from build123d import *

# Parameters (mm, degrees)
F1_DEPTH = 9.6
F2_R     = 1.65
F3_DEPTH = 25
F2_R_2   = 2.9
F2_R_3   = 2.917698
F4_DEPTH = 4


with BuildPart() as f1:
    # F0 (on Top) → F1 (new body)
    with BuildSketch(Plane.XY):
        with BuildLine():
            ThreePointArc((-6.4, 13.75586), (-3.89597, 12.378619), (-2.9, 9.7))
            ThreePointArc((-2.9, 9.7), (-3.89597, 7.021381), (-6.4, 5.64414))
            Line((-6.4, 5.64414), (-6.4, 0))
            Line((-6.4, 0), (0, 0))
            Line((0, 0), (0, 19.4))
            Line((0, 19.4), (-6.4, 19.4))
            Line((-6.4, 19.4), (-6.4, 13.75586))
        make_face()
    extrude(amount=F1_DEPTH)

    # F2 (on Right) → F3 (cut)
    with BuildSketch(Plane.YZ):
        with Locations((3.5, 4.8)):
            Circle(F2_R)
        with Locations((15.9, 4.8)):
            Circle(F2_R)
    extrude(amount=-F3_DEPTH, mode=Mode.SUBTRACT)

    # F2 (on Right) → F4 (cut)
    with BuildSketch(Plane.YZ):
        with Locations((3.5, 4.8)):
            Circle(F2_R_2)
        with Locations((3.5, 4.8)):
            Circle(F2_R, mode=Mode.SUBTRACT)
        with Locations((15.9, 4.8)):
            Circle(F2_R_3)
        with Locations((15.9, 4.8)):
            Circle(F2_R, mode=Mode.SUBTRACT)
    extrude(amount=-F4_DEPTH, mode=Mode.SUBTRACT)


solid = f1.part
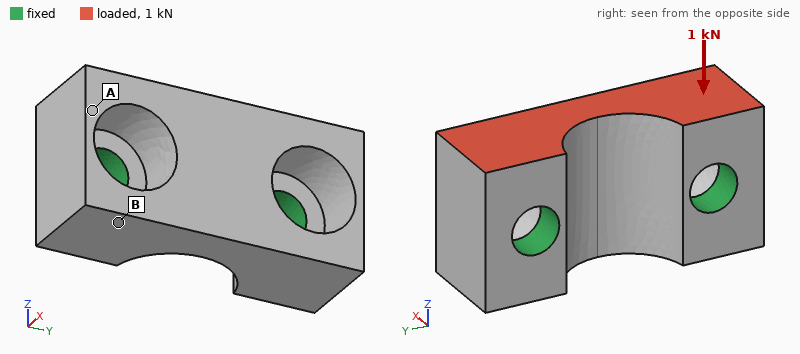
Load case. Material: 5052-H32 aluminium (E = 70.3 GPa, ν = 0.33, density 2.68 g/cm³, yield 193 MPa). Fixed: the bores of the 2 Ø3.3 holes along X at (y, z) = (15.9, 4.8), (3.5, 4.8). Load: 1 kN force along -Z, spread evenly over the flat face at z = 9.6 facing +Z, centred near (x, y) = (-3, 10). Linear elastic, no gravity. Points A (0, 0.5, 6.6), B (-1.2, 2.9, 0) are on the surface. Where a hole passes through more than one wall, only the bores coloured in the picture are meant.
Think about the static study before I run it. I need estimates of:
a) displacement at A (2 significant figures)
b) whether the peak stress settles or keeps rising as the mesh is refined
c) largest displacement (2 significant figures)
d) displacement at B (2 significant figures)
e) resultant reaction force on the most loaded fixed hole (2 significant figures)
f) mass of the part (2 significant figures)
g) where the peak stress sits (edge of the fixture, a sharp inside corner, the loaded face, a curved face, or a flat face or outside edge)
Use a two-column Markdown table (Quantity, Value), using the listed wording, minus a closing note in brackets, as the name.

| Quantity | Value |
|---|---|
| displacement at A | 7.3 µm |
| whether the peak stress settles or keeps rising as the mesh is refined | keeps rising |
| largest displacement | 11 µm |
| displacement at B | 6.2 µm |
| resultant reaction force on the most loaded fixed hole | 500 N |
| mass of the part | 2.0 g |
| where the peak stress sits | edge of the fixture |
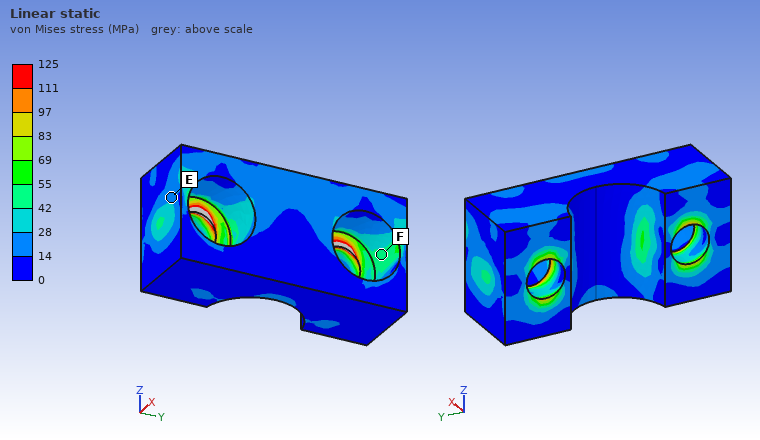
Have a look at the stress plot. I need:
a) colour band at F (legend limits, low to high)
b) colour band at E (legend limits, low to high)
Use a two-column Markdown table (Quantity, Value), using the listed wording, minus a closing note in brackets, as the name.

| Quantity | Value |
|---|---|
| colour band at F | 42 to 55 MPa |
| colour band at E | 14 to 28 MPa |
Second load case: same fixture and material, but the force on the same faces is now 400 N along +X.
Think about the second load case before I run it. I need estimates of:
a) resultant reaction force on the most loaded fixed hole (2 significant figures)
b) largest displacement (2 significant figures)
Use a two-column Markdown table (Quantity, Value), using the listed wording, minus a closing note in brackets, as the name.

| Quantity | Value |
|---|---|
| resultant reaction force on the most loaded fixed hole | 200 N |
| largest displacement | 7.2 µm |
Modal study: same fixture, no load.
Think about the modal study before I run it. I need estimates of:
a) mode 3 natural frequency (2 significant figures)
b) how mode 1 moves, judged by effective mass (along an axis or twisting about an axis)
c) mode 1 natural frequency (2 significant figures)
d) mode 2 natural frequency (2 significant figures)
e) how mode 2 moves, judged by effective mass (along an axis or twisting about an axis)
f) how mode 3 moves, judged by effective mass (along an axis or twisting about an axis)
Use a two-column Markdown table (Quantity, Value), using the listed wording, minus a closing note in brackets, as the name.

| Quantity | Value |
|---|---|
| mode 3 natural frequency | 67 kHz |
| how mode 1 moves, judged by effective mass | along Z |
| mode 1 natural frequency | 40 kHz |
| mode 2 natural frequency | 61 kHz |
| how mode 2 moves, judged by effective mass | twisting about X |
| how mode 3 moves, judged by effective mass | along Y |
